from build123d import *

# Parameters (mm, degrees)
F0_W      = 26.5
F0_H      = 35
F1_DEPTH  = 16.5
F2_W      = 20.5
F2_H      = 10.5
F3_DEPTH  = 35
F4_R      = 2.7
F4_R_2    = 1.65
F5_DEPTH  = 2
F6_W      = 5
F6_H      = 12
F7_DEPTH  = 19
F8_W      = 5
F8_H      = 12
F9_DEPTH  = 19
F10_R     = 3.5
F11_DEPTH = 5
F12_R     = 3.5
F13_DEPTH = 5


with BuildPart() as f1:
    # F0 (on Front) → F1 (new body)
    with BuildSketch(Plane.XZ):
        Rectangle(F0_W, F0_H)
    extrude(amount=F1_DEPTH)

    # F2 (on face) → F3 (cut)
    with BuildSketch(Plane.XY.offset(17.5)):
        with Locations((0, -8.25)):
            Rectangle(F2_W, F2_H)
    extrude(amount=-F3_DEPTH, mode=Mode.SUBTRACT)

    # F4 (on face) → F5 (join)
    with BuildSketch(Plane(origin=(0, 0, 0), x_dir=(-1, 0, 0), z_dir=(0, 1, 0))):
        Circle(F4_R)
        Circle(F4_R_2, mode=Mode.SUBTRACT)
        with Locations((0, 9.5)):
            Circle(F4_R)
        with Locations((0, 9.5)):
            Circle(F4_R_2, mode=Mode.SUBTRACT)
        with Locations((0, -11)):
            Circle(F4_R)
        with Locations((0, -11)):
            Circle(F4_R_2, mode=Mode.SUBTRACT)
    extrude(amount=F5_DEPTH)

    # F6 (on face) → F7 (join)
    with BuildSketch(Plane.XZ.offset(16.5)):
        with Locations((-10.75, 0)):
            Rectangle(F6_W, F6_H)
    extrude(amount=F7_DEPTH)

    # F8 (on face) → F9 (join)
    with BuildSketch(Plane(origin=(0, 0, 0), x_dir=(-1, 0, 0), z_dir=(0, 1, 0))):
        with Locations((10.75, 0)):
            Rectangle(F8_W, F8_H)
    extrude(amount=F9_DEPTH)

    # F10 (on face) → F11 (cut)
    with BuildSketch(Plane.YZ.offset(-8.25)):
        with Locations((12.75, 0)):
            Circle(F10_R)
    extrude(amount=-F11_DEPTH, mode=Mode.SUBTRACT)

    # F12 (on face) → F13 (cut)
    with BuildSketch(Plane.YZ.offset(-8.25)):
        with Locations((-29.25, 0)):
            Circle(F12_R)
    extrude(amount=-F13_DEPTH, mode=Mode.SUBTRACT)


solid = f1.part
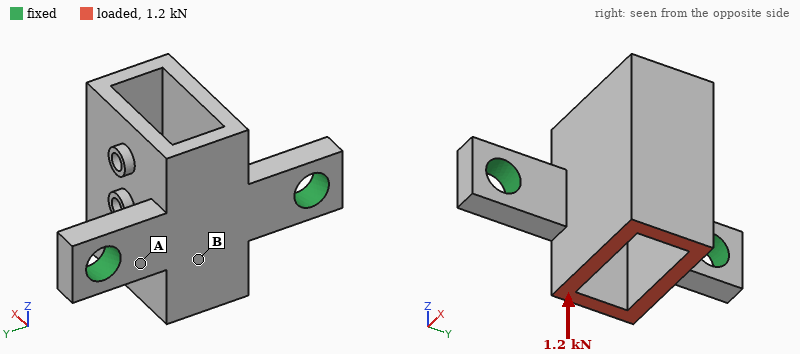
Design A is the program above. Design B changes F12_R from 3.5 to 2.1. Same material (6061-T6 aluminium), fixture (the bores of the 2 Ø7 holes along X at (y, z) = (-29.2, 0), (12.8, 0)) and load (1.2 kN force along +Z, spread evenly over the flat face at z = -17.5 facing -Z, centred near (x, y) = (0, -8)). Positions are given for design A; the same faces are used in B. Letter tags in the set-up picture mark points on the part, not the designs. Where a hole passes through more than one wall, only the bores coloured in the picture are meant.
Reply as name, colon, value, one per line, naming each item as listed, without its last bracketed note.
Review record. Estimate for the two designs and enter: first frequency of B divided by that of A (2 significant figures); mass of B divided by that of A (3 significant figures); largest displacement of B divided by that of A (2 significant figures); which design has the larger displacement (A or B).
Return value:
first frequency of B divided by that of A: 0.96
mass of B divided by that of A: 1.01
largest displacement of B divided by that of A: 1.1
which design has the larger displacement: B
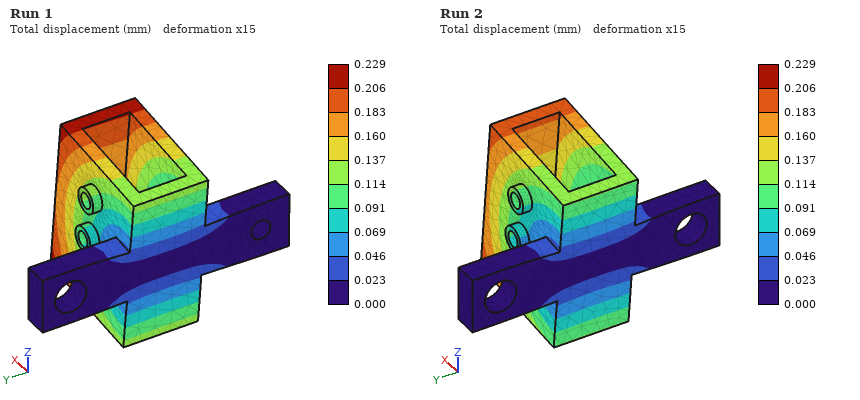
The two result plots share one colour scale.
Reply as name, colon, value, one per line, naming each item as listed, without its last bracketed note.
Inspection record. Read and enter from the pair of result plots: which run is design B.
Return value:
which run is design B: Run 1
